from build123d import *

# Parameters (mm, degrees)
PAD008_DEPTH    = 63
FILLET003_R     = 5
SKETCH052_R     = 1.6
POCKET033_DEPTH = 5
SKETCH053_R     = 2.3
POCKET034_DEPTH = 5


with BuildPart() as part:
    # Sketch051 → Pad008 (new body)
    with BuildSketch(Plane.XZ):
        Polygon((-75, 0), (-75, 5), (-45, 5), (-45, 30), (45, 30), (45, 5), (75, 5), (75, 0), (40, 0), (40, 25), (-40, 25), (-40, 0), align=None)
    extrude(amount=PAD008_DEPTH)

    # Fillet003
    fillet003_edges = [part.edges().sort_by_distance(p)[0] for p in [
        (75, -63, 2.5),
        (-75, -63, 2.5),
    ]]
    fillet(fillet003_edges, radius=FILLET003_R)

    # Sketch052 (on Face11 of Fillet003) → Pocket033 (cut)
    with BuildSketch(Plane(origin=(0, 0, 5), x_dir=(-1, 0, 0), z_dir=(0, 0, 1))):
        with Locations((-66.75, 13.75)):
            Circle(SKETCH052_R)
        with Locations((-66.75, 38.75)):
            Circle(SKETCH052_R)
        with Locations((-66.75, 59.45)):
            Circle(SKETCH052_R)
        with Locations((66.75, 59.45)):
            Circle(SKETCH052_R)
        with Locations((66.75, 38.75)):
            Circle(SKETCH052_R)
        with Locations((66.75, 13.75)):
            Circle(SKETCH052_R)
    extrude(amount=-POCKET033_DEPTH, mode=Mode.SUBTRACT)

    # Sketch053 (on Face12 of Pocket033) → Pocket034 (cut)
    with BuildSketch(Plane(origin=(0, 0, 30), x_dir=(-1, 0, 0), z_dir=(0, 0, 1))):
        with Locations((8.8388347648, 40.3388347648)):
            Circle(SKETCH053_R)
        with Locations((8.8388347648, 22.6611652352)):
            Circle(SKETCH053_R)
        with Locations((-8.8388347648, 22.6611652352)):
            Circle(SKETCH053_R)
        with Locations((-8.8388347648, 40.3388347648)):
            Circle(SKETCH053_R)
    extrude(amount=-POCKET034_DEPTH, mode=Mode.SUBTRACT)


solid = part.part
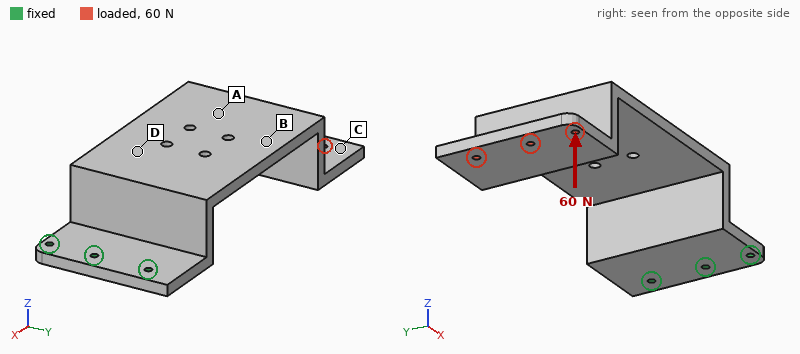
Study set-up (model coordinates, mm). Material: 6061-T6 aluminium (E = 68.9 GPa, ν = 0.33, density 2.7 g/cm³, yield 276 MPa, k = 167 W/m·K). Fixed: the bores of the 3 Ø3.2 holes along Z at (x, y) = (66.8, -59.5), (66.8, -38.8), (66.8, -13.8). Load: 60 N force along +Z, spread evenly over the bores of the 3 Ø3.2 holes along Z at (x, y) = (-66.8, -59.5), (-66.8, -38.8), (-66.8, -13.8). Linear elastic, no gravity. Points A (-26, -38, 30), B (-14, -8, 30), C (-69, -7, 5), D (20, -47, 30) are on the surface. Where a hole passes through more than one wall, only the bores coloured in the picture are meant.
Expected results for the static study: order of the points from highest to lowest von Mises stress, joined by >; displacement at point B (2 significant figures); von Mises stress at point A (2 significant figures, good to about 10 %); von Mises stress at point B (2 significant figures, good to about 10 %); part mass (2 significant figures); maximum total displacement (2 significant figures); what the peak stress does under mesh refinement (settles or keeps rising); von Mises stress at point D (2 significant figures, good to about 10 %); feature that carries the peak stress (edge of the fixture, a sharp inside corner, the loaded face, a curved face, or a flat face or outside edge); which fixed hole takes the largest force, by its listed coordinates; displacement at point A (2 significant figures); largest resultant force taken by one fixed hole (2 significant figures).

D > B > A > C
0.63 mm
8.3 MPa
13 MPa
170 g
1.5 mm
keeps rising
18 MPa
edge of the fixture
(66.8, -38.8)
0.80 mm
50 N
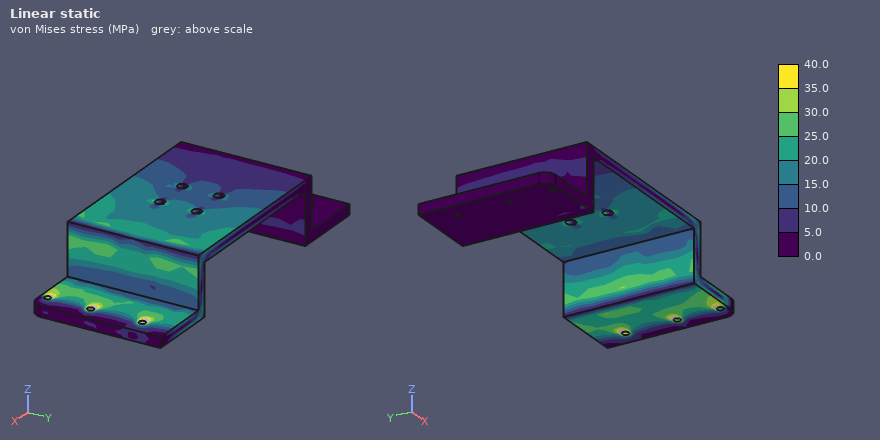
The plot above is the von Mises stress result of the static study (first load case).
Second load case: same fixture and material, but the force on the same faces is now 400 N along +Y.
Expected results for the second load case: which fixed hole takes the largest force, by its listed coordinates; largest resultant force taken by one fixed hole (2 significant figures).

(66.8, -13.8)
1.3 kN
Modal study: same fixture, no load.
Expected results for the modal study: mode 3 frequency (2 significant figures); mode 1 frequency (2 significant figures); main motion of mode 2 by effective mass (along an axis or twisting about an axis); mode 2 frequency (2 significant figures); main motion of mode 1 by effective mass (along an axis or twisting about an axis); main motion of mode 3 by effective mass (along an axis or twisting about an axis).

670 Hz
150 Hz
along Y
400 Hz
along Z
along X
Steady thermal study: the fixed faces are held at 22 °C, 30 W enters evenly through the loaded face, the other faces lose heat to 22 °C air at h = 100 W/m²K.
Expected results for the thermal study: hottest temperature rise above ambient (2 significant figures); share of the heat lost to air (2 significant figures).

36 K
91 %
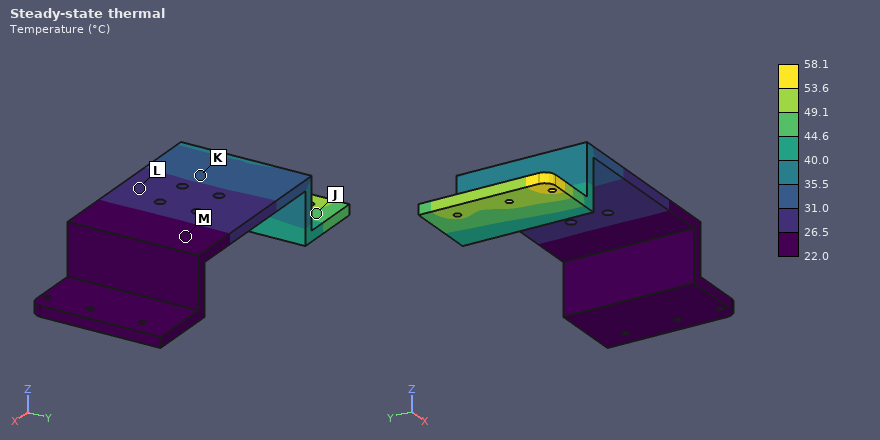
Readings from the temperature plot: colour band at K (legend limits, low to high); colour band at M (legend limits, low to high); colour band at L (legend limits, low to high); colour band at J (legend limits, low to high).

31.0 to 35.5 °C
22.0 to 26.5 °C
26.5 to 31.0 °C
44.6 to 49.1 °C
